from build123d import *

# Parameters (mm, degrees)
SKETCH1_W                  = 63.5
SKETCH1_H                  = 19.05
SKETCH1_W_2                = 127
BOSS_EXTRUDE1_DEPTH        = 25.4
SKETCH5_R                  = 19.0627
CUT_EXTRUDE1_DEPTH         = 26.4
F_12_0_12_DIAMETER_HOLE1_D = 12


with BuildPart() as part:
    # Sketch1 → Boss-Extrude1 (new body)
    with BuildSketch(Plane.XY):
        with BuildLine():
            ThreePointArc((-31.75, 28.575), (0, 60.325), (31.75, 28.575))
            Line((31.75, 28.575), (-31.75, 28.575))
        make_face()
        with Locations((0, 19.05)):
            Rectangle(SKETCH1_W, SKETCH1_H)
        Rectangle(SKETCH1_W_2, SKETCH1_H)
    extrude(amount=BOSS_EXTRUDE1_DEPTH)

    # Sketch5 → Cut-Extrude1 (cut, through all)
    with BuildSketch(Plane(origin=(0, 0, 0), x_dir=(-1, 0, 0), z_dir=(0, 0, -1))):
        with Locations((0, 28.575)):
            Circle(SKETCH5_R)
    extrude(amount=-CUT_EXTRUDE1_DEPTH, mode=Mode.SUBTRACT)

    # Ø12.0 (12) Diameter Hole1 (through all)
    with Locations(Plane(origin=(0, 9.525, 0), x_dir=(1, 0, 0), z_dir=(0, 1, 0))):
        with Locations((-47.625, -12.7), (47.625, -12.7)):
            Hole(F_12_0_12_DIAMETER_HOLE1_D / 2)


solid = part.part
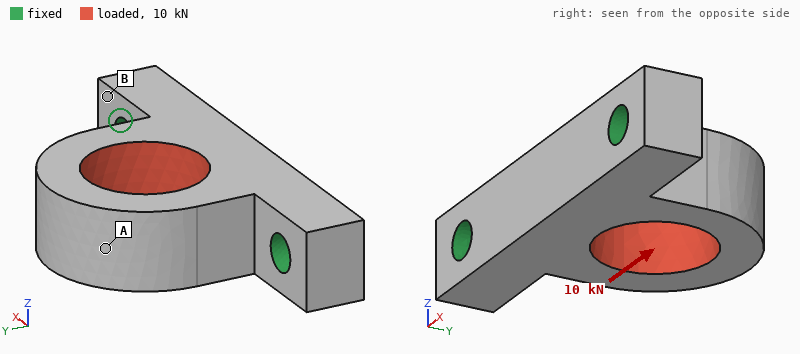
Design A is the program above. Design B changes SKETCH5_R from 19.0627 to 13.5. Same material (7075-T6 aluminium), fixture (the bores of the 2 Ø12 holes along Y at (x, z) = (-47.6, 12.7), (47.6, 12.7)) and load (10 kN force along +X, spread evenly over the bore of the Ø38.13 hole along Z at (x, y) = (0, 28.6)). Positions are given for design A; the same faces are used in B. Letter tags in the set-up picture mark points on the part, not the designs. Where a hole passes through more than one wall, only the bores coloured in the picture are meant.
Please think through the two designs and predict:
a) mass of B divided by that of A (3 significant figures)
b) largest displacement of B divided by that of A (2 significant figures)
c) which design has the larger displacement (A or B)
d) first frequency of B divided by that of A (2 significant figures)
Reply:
1.15
0.54
A
0.93
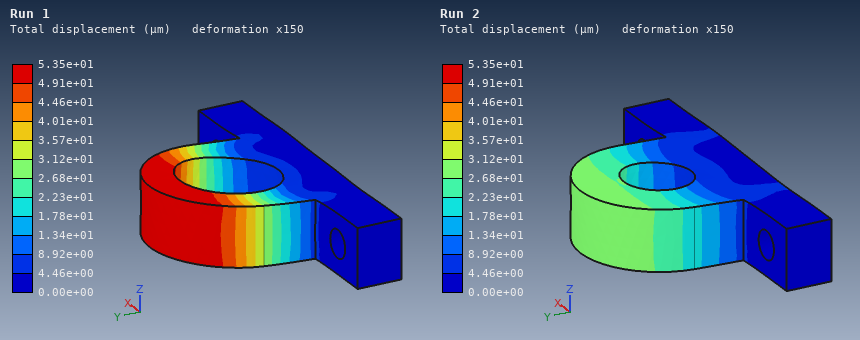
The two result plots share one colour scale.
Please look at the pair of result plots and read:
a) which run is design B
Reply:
Run 2
